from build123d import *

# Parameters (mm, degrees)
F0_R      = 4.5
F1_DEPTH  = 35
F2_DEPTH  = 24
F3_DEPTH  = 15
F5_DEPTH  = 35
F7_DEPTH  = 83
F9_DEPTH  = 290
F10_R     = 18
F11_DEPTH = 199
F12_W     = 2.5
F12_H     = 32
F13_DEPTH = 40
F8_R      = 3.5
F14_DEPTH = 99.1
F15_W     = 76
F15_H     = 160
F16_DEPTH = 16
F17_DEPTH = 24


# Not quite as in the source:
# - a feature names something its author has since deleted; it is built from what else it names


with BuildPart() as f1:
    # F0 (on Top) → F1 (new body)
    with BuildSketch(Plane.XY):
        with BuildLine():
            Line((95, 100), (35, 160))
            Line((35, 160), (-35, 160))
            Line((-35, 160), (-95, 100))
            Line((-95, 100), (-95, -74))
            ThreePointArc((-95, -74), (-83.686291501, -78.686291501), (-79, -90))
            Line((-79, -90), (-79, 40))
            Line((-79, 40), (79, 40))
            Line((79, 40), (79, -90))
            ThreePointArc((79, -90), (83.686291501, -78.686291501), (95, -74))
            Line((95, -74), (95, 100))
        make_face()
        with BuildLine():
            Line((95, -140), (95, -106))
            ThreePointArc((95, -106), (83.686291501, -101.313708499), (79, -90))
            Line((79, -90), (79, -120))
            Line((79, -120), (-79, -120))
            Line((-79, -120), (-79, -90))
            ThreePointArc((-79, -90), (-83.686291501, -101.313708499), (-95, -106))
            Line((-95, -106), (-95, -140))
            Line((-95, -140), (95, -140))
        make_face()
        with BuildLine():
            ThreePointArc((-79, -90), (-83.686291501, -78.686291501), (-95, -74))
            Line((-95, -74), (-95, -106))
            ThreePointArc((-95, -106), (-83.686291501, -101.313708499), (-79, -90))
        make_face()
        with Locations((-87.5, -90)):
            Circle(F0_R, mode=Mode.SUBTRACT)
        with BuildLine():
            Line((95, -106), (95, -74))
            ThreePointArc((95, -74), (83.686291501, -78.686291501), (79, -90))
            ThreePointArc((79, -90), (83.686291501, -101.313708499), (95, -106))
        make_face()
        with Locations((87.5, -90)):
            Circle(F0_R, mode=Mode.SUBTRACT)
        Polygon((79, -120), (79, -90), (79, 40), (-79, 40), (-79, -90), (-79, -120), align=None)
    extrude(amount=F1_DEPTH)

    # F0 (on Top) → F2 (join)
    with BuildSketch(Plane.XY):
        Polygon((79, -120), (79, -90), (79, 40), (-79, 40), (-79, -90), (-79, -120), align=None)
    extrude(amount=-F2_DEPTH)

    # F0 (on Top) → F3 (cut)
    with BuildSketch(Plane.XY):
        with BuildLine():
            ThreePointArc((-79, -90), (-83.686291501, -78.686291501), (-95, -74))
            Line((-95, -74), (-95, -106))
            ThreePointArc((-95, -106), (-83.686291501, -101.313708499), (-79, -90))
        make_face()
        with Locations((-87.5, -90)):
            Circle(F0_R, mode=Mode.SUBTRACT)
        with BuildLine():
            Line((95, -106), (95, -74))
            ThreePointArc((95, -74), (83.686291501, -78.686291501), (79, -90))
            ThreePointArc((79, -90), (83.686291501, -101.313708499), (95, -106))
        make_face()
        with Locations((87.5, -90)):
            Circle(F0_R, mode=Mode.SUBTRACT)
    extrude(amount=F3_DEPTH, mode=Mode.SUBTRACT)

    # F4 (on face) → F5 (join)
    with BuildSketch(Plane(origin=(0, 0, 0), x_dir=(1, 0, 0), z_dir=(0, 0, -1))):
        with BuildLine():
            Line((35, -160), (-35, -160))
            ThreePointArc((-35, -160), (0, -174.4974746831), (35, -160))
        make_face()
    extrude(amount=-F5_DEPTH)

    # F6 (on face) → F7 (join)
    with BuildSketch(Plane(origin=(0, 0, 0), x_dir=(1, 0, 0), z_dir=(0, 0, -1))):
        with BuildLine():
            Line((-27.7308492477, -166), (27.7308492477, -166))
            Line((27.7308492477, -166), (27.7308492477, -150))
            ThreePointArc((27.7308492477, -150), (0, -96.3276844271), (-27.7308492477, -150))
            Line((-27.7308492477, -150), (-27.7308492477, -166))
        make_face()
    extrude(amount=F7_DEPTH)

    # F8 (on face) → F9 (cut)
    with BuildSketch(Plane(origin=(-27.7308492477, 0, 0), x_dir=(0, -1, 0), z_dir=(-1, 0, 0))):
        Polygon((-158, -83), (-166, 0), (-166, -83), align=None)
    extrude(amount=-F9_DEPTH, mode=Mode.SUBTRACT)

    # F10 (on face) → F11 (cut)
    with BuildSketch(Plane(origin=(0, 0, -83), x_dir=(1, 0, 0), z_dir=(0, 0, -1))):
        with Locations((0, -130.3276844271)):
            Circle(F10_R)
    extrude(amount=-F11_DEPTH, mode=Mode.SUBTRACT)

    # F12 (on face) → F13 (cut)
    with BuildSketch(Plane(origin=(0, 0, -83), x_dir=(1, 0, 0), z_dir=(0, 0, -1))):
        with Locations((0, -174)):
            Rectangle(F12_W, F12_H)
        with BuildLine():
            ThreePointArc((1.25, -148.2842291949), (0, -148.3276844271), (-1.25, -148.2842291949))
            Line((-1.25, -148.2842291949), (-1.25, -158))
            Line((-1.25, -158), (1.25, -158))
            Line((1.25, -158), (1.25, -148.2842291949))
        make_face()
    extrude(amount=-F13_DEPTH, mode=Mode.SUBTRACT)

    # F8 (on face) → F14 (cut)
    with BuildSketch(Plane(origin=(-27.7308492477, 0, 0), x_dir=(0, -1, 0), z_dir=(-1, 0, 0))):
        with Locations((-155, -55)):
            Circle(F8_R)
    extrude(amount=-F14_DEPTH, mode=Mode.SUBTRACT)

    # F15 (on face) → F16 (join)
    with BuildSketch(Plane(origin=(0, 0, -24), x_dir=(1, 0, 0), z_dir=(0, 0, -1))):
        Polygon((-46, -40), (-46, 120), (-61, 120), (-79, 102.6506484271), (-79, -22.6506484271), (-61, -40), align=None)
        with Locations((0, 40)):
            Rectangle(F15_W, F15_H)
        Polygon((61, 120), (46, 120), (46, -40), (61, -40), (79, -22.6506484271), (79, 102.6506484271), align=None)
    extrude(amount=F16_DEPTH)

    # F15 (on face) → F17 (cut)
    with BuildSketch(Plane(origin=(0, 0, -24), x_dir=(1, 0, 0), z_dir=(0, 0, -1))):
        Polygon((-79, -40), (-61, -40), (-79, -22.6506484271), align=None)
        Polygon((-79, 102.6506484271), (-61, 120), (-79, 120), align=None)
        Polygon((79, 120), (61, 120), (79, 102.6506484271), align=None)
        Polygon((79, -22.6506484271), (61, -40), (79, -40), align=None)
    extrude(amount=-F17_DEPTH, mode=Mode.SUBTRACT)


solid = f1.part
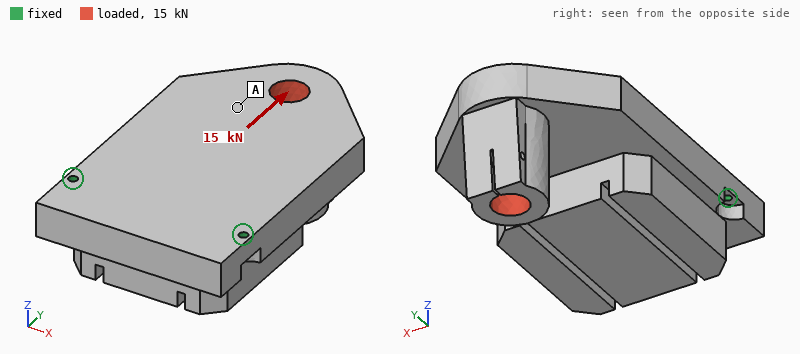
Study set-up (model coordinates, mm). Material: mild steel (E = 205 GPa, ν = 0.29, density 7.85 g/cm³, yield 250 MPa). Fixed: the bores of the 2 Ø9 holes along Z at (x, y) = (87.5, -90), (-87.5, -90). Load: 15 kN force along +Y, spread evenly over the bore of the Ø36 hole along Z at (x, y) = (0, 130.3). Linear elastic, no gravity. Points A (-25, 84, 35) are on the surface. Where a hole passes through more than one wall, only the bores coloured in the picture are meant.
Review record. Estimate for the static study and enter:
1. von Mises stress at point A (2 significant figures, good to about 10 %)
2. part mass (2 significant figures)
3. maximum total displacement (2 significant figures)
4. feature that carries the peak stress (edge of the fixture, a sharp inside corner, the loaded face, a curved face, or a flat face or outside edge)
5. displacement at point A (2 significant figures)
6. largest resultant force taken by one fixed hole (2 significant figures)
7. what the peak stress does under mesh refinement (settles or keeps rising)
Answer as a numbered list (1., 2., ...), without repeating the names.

1. 14 MPa
2. 24 kg
3. 0.28 mm
4. edge of the fixture
5. 0.14 mm
6. 7.5 kN
7. keeps rising
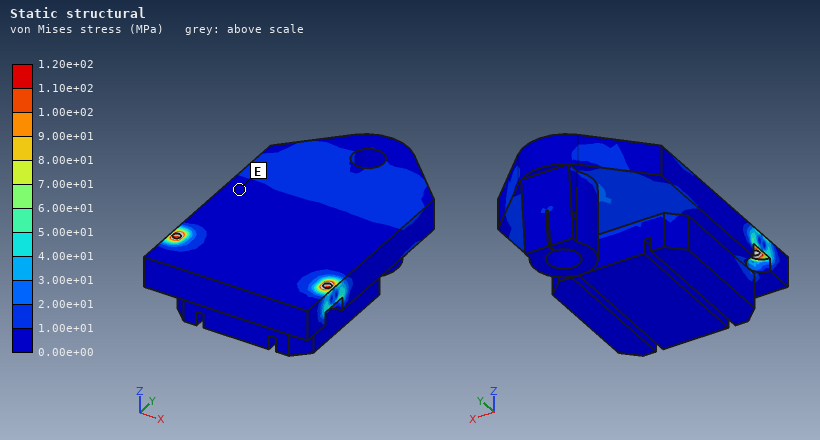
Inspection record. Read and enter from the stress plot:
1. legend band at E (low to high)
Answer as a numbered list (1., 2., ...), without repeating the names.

1. 0.00e+00 to 1.00e+01 MPa
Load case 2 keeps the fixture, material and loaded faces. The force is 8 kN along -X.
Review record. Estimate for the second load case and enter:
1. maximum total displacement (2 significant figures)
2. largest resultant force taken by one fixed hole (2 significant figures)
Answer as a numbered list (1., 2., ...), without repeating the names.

1. 37 µm
2. 11 kN
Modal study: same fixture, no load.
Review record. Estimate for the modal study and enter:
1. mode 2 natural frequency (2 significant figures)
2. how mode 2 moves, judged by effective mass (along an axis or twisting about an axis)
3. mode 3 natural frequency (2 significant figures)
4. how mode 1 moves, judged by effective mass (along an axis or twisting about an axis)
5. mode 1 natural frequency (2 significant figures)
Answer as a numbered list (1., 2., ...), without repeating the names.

1. 1400 Hz
2. along X
3. 1600 Hz
4. along Z
5. 250 Hz
